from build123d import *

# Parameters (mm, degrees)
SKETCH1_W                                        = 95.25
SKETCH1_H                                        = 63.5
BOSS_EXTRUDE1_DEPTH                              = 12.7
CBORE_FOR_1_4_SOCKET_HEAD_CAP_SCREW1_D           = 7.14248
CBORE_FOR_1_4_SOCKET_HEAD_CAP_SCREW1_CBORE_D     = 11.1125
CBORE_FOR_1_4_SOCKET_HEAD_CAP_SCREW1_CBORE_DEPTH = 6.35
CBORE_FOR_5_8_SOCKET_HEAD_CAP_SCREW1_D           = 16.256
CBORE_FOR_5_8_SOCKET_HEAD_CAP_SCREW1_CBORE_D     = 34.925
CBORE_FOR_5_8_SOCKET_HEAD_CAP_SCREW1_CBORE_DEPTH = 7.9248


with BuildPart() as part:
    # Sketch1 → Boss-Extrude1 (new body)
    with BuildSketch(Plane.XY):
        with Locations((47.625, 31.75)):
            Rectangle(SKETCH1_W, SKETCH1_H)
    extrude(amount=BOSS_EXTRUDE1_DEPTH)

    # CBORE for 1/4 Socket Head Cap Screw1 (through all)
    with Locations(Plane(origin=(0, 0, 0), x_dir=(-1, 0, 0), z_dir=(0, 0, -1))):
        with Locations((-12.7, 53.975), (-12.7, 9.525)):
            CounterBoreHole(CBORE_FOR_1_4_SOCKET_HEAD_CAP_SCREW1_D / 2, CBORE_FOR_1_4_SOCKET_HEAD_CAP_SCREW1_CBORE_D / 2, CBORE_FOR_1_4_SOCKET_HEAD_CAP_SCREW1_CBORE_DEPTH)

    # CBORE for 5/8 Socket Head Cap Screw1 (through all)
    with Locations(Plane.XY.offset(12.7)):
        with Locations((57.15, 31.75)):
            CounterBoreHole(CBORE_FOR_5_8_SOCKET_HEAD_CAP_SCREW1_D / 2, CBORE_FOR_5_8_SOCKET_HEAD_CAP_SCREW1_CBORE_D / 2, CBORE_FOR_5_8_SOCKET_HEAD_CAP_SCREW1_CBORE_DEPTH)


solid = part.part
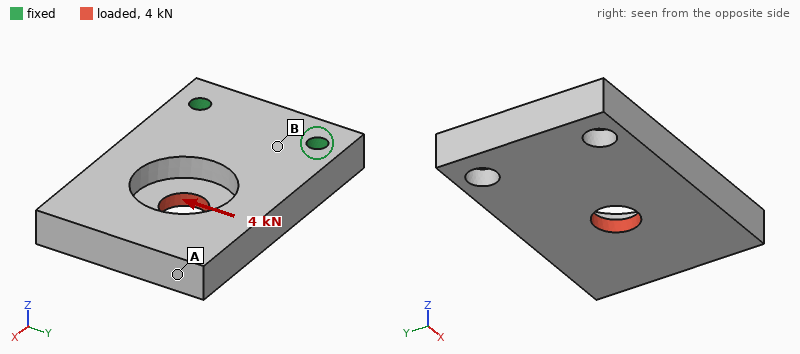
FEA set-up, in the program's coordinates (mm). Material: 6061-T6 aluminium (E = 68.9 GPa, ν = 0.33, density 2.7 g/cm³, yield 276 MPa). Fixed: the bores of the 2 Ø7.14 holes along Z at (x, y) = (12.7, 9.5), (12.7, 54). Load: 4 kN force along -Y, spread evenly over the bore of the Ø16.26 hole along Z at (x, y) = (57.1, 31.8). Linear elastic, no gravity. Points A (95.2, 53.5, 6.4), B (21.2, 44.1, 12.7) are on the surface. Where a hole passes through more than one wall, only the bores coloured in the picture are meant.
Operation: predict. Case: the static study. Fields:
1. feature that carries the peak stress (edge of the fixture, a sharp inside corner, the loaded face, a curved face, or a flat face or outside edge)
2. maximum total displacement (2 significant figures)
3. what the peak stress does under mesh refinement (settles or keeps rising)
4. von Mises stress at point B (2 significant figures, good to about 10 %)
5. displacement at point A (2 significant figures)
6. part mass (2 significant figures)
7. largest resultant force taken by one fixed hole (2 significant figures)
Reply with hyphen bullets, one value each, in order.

- edge of the fixture
- 42 µm
- keeps rising
- 18 MPa
- 41 µm
- 180 g
- 4.3 kN
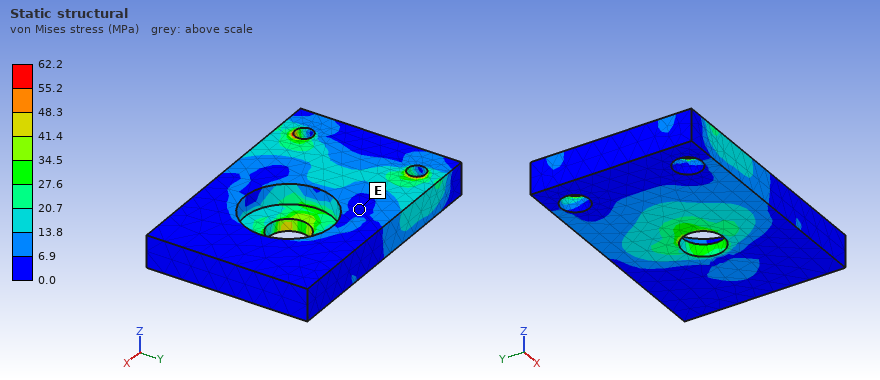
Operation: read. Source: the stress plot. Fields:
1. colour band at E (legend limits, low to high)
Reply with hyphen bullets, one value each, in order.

- 0.0 to 6.9 MPa
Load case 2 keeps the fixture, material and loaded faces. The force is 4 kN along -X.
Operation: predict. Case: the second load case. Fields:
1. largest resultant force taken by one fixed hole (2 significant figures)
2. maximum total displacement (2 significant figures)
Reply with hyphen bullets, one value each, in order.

- 2.0 kN
- 0.13 mm
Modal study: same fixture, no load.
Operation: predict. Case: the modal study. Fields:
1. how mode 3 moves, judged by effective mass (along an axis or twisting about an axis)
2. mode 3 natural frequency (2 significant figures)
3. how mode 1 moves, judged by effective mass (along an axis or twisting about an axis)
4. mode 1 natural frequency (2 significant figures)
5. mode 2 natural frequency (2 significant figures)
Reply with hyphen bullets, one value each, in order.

- along Y
- 4800 Hz
- along Z
- 1100 Hz
- 3300 Hz
